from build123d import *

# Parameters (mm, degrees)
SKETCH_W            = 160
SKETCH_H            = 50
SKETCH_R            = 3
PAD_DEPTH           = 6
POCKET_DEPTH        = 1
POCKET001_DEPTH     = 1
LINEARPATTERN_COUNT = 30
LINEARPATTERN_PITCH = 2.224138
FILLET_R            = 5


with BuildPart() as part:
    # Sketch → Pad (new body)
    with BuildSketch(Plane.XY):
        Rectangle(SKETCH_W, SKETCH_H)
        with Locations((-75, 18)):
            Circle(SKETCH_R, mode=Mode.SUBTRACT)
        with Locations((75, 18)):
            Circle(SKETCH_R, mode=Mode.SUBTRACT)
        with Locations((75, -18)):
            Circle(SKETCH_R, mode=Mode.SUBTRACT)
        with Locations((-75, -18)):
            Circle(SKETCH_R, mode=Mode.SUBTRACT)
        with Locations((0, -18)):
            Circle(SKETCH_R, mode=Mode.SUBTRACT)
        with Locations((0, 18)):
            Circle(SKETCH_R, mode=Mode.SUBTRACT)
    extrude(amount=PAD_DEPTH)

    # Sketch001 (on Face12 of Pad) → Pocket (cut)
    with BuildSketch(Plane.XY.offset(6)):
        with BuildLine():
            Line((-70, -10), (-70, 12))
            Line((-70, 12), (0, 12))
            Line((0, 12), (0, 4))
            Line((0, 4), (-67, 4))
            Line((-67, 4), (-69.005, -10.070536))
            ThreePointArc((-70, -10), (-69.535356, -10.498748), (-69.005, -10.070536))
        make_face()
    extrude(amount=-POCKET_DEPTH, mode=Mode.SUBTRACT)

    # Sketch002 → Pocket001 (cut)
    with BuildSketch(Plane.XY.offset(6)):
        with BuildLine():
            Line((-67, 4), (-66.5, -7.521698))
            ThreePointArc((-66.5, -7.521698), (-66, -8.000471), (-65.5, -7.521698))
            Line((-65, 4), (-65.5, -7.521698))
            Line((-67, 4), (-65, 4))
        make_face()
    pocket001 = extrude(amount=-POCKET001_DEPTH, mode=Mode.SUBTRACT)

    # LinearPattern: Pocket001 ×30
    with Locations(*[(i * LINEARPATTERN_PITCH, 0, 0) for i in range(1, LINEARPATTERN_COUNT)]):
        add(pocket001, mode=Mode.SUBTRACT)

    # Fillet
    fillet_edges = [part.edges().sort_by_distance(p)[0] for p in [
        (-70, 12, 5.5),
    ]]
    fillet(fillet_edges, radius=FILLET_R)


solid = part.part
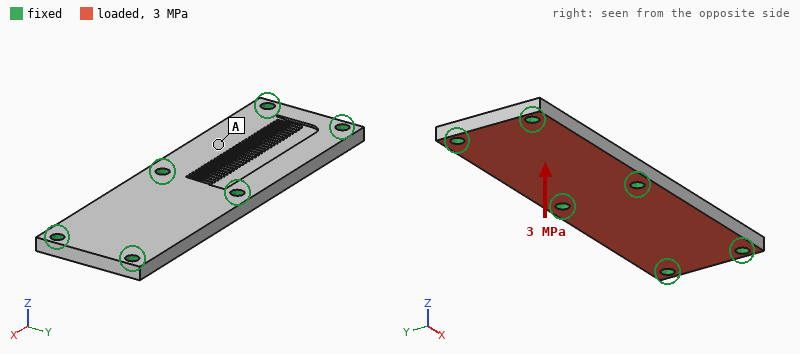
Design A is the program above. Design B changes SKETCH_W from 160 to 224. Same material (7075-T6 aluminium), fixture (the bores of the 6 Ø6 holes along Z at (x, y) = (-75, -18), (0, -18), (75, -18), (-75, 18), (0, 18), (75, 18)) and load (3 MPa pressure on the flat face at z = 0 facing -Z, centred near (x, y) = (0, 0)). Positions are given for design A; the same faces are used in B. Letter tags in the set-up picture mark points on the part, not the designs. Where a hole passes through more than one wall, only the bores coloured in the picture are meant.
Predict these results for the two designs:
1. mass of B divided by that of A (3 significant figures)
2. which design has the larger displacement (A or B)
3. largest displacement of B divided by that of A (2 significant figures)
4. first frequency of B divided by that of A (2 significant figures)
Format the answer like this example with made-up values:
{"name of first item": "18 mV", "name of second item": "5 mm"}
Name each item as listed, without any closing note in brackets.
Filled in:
{"mass of B divided by that of A": "1.42", "which design has the larger displacement": "B", "largest displacement of B divided by that of A": "2.4", "first frequency of B divided by that of A": "0.68"}
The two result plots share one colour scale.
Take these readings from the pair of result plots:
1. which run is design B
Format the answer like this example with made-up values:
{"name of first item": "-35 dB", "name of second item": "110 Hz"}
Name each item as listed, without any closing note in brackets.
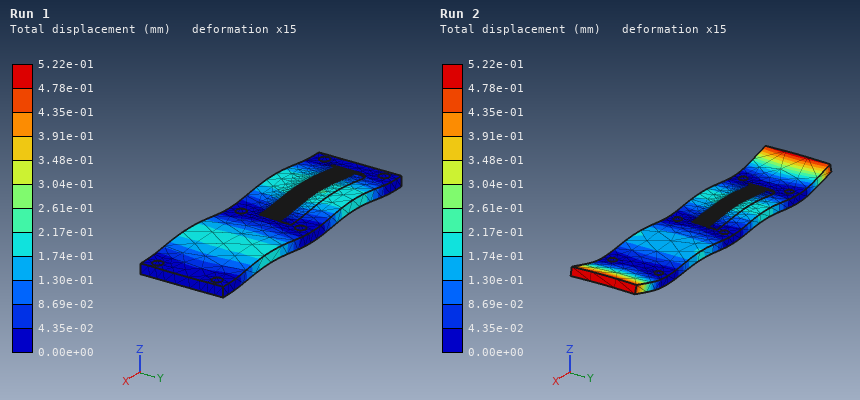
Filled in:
{"which run is design B": "Run 2"}
